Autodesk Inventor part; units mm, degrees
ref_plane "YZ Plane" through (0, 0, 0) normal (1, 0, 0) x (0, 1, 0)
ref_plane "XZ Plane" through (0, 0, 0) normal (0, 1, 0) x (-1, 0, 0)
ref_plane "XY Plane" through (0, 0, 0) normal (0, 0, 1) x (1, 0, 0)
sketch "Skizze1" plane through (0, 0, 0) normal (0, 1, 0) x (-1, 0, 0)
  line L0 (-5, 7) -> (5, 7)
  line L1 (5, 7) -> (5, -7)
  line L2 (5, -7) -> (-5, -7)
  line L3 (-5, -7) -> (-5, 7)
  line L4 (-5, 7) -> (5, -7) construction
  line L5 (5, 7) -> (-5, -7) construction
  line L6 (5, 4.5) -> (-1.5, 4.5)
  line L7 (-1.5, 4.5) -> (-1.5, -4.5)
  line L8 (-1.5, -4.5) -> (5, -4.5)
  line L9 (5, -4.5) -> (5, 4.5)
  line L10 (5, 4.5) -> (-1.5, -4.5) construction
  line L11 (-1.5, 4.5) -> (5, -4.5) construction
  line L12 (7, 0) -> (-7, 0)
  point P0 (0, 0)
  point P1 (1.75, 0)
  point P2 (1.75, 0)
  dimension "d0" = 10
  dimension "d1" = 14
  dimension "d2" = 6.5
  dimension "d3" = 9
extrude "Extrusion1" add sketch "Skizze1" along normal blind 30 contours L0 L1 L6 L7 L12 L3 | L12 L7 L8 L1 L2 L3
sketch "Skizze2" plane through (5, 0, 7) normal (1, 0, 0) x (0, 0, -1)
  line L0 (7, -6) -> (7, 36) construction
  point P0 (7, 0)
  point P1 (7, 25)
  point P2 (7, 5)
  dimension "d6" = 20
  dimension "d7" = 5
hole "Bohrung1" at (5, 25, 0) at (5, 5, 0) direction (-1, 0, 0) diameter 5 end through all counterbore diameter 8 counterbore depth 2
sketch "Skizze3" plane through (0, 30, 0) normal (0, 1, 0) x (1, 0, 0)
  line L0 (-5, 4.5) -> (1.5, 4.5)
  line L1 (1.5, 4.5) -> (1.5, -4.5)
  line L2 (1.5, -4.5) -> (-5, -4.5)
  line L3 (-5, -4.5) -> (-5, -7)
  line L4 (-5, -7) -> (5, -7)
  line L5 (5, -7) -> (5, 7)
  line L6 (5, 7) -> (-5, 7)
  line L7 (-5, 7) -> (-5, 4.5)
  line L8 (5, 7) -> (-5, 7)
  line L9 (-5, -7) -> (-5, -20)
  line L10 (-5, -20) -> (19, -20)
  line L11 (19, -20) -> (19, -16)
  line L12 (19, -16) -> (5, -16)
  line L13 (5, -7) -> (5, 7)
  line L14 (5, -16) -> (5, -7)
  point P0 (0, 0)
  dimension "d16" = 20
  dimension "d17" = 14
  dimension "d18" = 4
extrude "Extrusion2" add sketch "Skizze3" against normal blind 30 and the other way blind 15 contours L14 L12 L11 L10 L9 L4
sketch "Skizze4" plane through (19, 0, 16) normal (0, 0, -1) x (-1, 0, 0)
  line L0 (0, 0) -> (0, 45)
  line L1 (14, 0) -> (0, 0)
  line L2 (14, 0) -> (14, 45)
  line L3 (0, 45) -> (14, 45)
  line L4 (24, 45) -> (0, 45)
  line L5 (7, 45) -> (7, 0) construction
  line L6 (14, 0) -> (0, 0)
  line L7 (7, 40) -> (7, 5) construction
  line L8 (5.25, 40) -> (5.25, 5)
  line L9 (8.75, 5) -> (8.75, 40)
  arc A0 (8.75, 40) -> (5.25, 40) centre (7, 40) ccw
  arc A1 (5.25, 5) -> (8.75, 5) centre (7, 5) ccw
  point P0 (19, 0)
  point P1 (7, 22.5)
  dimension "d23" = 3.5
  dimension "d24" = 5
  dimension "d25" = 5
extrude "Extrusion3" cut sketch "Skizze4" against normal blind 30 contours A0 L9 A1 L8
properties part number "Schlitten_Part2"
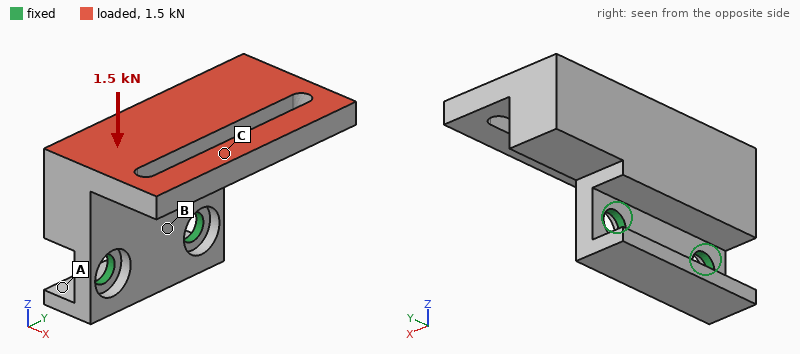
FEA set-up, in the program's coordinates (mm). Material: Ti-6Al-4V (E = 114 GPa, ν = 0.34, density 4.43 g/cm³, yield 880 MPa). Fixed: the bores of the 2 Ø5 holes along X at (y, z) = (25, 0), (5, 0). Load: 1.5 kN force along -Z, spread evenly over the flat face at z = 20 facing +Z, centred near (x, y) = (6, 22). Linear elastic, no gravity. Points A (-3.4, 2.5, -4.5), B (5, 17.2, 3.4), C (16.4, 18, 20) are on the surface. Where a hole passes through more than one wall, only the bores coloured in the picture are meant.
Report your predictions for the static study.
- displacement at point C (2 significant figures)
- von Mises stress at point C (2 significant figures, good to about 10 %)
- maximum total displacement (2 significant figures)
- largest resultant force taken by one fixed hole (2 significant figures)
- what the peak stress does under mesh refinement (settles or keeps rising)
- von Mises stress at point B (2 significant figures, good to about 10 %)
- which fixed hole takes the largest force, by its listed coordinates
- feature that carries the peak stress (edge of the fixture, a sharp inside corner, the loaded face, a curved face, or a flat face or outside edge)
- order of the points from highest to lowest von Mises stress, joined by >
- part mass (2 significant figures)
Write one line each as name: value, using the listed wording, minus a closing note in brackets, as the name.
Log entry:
displacement at point C: 0.20 mm
von Mises stress at point C: 67 MPa
maximum total displacement: 0.23 mm
largest resultant force taken by one fixed hole: 1.3 kN
what the peak stress does under mesh refinement: keeps rising
von Mises stress at point B: 99 MPa
which fixed hole takes the largest force, by its listed coordinates: (25, 0)
feature that carries the peak stress: edge of the fixture
order of the points from highest to lowest von Mises stress, joined by >: B > C > A
part mass: 44 g
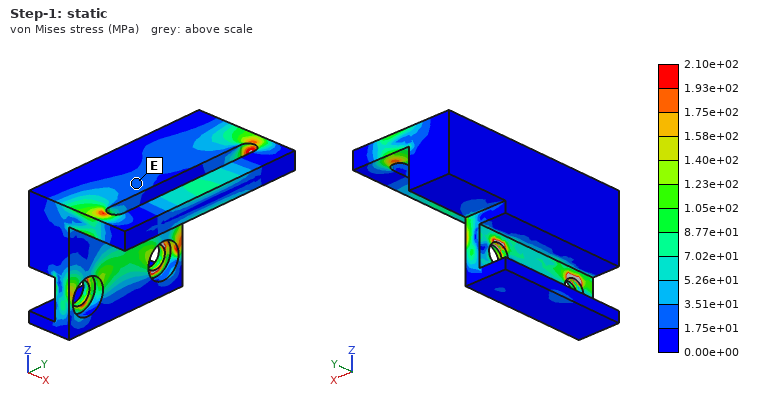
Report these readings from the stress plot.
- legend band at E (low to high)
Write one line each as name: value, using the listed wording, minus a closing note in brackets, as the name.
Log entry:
legend band at E: 1.75e+01 to 3.51e+01 MPa
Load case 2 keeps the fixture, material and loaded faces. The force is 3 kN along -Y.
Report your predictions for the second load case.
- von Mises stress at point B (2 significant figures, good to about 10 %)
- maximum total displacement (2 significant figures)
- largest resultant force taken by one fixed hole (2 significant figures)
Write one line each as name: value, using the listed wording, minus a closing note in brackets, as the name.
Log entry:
von Mises stress at point B: 67 MPa
maximum total displacement: 92 µm
largest resultant force taken by one fixed hole: 3.1 kN
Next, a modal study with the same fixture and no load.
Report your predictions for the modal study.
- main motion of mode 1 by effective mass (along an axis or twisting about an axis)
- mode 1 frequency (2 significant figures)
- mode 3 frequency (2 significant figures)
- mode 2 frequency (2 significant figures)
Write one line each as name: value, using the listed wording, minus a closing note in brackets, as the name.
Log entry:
main motion of mode 1 by effective mass: along X
mode 1 frequency: 2000 Hz
mode 3 frequency: 6300 Hz
mode 2 frequency: 5300 Hz
